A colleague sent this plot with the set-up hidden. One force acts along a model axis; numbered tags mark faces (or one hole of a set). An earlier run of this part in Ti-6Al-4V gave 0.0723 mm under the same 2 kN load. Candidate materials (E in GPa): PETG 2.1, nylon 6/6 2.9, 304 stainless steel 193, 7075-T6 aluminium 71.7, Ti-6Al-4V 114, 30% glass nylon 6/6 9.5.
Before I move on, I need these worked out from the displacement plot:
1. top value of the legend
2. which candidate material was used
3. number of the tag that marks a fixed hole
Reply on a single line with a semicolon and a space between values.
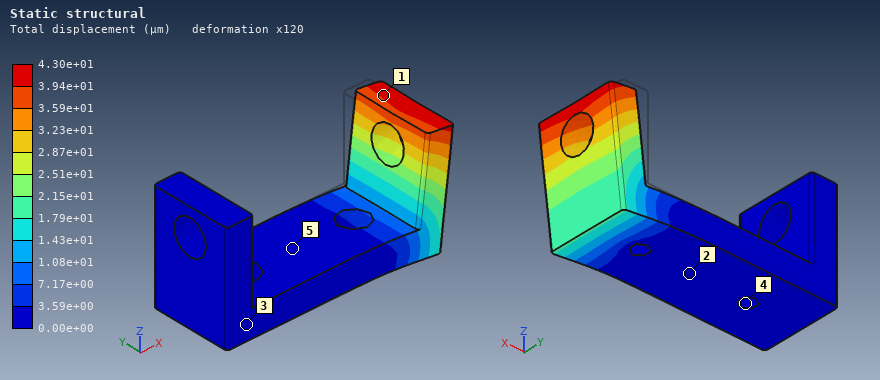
4.30e+01 µm; 304 stainless steel; 4
